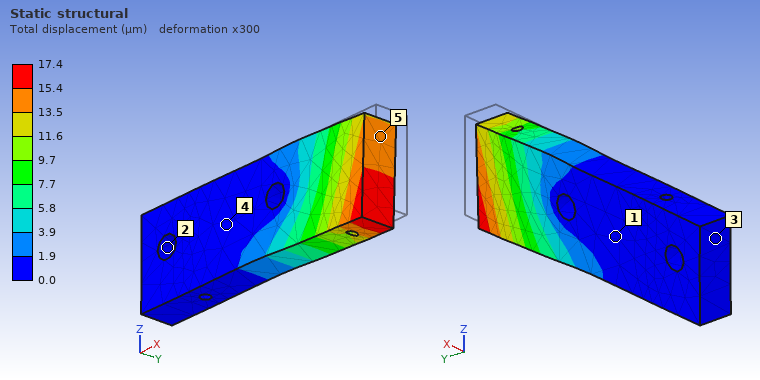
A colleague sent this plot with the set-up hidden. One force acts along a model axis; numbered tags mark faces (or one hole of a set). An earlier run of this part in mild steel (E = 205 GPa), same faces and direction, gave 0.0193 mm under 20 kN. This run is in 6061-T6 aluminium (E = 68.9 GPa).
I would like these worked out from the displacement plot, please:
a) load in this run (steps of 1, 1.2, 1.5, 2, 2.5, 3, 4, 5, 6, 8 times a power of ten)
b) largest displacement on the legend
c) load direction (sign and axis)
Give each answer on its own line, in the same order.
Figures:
6 kN
17.4 µm
-X
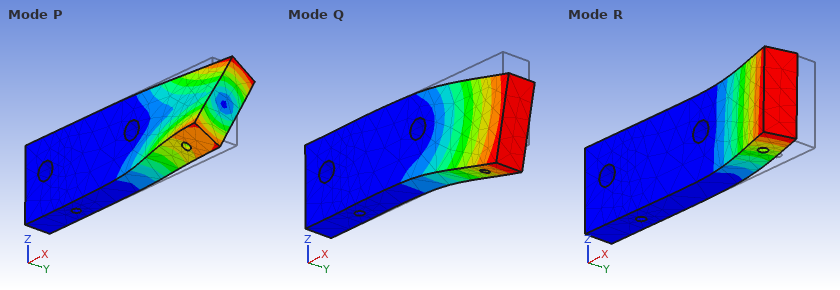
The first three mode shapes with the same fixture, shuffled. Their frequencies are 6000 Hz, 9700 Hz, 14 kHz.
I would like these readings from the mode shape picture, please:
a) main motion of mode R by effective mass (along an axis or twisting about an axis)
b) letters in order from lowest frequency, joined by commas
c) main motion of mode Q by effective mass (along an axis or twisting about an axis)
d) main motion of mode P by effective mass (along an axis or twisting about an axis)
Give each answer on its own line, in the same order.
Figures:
along Y
R, Q, P
along Z
twisting about X
